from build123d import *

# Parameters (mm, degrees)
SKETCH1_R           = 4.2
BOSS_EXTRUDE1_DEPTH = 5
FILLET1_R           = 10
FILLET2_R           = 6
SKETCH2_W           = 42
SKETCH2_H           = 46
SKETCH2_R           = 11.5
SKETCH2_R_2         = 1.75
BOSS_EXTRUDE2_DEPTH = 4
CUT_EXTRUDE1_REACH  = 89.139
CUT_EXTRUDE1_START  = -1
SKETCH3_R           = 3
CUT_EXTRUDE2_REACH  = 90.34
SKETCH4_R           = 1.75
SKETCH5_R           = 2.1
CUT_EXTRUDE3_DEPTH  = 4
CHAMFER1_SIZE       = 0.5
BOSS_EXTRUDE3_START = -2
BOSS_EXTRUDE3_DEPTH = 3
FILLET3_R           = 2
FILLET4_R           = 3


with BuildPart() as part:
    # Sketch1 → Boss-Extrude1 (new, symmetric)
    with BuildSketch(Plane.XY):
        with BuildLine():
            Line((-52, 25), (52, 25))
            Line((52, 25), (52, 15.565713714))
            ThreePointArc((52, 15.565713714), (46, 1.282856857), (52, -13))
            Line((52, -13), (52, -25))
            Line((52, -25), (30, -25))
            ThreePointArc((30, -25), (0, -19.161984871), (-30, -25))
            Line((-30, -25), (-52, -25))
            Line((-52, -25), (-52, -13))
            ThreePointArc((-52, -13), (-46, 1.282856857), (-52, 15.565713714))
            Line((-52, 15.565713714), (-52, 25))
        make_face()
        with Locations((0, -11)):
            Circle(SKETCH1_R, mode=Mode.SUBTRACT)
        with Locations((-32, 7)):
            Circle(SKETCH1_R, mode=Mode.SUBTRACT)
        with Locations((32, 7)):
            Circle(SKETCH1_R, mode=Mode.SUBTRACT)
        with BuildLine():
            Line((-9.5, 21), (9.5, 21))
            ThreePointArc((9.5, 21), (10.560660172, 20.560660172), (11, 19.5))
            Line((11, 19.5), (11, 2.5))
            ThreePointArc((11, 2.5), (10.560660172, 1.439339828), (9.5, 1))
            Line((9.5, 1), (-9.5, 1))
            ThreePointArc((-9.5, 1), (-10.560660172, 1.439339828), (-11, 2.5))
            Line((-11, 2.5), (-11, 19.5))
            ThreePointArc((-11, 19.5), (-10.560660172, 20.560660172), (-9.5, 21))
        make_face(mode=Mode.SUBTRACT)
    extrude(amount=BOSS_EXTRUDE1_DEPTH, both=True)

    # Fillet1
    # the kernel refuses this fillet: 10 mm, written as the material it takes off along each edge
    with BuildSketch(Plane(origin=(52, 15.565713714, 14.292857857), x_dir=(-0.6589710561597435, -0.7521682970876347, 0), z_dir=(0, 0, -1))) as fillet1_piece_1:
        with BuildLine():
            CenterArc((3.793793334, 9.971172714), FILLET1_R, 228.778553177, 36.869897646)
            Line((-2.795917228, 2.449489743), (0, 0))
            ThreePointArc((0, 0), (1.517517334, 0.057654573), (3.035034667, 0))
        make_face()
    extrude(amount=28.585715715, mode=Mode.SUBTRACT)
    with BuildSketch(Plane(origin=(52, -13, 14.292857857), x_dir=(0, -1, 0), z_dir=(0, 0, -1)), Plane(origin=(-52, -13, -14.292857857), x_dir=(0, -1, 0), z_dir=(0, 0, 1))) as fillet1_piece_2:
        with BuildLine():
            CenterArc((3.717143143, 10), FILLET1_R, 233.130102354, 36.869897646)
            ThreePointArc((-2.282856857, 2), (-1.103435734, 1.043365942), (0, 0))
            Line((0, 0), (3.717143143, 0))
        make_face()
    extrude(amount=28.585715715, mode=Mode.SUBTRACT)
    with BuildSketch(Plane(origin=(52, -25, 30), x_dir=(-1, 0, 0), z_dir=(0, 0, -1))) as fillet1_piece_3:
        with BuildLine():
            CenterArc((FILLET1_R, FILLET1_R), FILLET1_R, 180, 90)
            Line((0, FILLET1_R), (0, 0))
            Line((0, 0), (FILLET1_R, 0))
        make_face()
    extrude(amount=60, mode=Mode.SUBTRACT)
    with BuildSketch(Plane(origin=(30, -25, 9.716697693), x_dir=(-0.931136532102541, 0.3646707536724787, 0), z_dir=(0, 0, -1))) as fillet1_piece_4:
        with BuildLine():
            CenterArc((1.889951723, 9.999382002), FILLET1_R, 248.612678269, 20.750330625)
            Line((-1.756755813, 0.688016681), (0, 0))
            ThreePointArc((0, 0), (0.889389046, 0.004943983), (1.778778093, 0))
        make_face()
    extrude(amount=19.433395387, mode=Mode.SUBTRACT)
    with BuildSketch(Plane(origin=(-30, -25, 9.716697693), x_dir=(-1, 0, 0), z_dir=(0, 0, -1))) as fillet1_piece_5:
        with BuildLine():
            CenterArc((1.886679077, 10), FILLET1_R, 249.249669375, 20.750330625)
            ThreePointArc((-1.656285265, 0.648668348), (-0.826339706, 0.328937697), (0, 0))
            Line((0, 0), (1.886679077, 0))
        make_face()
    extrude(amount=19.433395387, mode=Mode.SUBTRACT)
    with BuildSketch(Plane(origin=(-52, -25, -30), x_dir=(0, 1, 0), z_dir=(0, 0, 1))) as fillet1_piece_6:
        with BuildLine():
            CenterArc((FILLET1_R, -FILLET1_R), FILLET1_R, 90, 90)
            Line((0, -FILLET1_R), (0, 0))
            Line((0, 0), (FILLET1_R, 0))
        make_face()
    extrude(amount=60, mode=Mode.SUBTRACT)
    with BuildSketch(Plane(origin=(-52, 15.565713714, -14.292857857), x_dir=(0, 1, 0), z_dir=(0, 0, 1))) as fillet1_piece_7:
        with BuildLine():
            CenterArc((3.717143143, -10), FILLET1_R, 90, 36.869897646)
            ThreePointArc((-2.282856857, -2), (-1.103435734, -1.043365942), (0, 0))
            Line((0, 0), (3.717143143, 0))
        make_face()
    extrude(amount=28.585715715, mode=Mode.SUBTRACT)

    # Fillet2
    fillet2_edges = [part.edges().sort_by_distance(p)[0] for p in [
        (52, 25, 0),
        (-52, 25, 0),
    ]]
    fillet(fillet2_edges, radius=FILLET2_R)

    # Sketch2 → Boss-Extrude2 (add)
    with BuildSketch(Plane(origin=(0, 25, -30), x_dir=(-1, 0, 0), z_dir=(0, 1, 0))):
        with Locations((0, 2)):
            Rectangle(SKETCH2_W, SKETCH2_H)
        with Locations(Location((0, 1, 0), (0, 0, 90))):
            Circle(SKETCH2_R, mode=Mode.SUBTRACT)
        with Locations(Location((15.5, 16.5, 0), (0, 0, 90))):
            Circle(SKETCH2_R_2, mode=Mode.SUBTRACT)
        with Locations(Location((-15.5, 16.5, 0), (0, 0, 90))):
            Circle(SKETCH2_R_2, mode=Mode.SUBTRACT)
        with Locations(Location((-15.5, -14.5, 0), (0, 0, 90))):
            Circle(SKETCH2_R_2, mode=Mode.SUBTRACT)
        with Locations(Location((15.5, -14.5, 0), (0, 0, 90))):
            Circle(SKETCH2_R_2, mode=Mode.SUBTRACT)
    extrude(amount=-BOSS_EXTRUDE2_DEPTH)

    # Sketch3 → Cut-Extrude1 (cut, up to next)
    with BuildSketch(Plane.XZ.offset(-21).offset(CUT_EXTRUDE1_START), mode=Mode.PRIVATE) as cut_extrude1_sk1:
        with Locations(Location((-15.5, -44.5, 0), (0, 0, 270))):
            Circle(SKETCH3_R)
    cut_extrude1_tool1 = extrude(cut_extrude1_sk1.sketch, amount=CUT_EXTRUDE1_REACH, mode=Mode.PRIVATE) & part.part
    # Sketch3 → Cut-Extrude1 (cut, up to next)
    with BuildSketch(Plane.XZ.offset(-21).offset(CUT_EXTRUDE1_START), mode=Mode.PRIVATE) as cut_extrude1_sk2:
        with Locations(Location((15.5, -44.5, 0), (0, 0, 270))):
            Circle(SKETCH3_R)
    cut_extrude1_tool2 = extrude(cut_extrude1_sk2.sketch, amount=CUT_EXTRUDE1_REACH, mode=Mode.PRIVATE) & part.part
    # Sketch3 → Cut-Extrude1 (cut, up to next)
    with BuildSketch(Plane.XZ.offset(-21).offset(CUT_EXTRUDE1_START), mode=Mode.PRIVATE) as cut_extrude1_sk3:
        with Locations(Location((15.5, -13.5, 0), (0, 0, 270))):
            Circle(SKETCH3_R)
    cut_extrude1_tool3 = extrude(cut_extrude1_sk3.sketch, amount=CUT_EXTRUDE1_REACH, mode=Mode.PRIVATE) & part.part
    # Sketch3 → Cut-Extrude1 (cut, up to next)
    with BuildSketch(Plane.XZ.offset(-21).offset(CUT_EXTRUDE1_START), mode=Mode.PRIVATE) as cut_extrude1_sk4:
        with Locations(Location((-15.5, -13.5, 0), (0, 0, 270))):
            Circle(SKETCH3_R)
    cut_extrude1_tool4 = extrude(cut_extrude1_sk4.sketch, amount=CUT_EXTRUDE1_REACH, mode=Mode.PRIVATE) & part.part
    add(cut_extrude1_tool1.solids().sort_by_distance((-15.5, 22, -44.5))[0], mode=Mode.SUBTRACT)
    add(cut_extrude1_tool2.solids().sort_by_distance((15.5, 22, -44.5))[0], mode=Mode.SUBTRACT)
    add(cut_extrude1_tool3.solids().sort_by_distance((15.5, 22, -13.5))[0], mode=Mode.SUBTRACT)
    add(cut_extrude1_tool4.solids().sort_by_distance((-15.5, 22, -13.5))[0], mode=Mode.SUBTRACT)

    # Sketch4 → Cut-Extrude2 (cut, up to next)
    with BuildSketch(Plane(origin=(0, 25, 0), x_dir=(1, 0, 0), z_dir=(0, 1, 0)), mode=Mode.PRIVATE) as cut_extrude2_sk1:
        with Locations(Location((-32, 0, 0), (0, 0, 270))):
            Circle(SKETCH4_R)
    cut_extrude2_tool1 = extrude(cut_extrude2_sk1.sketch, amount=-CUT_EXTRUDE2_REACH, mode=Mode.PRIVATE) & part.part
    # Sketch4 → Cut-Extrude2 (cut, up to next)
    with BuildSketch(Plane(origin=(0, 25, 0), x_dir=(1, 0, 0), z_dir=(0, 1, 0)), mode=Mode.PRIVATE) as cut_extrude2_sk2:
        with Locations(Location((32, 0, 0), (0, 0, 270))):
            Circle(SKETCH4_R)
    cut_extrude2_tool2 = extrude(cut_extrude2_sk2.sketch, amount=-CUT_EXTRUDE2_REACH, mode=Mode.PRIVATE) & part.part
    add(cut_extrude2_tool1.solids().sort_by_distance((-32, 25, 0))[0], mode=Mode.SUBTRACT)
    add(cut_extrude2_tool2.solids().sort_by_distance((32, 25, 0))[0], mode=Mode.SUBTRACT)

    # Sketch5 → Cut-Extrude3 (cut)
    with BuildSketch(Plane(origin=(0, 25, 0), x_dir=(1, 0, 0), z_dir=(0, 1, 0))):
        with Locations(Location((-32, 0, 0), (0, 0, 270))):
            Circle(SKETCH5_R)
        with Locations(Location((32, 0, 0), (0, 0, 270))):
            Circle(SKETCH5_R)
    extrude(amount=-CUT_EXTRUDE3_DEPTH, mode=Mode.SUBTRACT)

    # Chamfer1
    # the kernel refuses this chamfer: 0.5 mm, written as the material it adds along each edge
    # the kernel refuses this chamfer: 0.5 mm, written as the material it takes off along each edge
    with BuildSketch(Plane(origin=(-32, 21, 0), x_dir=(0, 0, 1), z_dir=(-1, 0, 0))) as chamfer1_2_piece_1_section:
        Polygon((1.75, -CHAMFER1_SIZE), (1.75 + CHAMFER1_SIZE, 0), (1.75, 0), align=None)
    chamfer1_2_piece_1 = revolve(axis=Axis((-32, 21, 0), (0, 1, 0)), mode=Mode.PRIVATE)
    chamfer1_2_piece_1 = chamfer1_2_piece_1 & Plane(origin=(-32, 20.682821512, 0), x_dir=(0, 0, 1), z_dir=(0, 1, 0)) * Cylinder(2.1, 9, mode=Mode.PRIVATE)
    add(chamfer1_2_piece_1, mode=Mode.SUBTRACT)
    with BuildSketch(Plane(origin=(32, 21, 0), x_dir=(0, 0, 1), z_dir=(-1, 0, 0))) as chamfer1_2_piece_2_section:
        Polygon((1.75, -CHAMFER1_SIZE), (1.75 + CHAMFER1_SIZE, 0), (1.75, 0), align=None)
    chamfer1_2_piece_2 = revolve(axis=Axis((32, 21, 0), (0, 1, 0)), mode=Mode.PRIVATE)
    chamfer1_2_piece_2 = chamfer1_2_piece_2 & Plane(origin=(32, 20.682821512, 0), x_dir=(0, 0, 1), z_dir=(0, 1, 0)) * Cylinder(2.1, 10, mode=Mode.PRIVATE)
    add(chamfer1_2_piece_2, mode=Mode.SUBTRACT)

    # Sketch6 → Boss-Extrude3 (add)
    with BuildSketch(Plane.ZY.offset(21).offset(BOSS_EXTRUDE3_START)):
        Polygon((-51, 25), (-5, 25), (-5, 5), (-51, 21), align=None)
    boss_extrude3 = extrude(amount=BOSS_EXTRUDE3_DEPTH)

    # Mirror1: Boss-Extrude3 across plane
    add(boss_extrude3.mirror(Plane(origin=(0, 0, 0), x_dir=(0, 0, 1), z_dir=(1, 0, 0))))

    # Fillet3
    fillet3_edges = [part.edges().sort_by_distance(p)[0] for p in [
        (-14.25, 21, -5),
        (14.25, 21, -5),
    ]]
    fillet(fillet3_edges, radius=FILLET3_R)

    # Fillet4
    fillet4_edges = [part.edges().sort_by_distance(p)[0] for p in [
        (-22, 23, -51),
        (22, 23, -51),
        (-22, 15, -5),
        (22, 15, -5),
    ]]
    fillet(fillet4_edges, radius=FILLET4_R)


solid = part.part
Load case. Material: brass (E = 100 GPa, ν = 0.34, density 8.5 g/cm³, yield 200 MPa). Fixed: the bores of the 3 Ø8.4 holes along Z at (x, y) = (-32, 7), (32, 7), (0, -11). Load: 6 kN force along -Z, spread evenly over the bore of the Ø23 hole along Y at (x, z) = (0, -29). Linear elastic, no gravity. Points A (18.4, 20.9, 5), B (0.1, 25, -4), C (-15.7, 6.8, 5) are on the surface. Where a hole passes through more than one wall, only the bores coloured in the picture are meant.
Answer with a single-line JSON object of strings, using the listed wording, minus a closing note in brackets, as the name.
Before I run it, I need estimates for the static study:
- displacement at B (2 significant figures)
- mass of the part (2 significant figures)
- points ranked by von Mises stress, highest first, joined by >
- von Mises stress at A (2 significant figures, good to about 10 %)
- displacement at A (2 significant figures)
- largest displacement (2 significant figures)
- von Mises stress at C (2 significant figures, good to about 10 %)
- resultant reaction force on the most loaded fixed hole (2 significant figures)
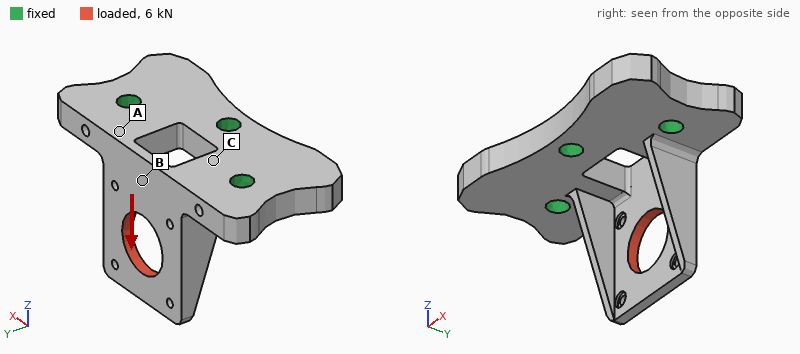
{"displacement at B": "0.050 mm", "mass of the part": "410 g", "points ranked by von Mises stress, highest first, joined by >": "C > A > B", "von Mises stress at A": "28 MPa", "displacement at A": "0.031 mm", "largest displacement": "0.16 mm", "von Mises stress at C": "42 MPa", "resultant reaction force on the most loaded fixed hole": "3.2 kN"}
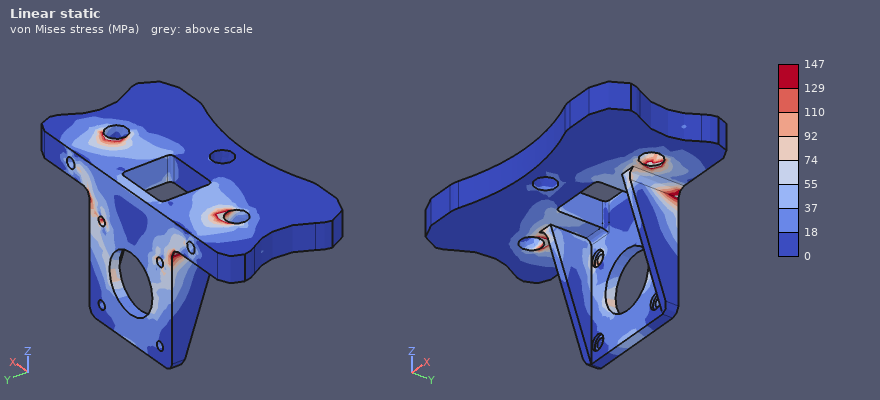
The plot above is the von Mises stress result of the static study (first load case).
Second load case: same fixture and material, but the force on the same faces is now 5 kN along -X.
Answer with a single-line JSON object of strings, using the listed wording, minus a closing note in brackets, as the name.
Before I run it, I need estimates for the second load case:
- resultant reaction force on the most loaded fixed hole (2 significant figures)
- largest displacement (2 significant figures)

{"resultant reaction force on the most loaded fixed hole": "4.0 kN", "largest displacement": "0.17 mm"}
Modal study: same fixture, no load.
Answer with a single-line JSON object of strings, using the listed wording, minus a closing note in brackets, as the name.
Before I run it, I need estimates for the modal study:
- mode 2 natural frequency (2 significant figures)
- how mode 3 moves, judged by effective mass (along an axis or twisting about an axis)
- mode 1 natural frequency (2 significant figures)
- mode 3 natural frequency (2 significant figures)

{"mode 2 natural frequency": "3500 Hz", "how mode 3 moves, judged by effective mass": "twisting about X", "mode 1 natural frequency": "2400 Hz", "mode 3 natural frequency": "6100 Hz"}
